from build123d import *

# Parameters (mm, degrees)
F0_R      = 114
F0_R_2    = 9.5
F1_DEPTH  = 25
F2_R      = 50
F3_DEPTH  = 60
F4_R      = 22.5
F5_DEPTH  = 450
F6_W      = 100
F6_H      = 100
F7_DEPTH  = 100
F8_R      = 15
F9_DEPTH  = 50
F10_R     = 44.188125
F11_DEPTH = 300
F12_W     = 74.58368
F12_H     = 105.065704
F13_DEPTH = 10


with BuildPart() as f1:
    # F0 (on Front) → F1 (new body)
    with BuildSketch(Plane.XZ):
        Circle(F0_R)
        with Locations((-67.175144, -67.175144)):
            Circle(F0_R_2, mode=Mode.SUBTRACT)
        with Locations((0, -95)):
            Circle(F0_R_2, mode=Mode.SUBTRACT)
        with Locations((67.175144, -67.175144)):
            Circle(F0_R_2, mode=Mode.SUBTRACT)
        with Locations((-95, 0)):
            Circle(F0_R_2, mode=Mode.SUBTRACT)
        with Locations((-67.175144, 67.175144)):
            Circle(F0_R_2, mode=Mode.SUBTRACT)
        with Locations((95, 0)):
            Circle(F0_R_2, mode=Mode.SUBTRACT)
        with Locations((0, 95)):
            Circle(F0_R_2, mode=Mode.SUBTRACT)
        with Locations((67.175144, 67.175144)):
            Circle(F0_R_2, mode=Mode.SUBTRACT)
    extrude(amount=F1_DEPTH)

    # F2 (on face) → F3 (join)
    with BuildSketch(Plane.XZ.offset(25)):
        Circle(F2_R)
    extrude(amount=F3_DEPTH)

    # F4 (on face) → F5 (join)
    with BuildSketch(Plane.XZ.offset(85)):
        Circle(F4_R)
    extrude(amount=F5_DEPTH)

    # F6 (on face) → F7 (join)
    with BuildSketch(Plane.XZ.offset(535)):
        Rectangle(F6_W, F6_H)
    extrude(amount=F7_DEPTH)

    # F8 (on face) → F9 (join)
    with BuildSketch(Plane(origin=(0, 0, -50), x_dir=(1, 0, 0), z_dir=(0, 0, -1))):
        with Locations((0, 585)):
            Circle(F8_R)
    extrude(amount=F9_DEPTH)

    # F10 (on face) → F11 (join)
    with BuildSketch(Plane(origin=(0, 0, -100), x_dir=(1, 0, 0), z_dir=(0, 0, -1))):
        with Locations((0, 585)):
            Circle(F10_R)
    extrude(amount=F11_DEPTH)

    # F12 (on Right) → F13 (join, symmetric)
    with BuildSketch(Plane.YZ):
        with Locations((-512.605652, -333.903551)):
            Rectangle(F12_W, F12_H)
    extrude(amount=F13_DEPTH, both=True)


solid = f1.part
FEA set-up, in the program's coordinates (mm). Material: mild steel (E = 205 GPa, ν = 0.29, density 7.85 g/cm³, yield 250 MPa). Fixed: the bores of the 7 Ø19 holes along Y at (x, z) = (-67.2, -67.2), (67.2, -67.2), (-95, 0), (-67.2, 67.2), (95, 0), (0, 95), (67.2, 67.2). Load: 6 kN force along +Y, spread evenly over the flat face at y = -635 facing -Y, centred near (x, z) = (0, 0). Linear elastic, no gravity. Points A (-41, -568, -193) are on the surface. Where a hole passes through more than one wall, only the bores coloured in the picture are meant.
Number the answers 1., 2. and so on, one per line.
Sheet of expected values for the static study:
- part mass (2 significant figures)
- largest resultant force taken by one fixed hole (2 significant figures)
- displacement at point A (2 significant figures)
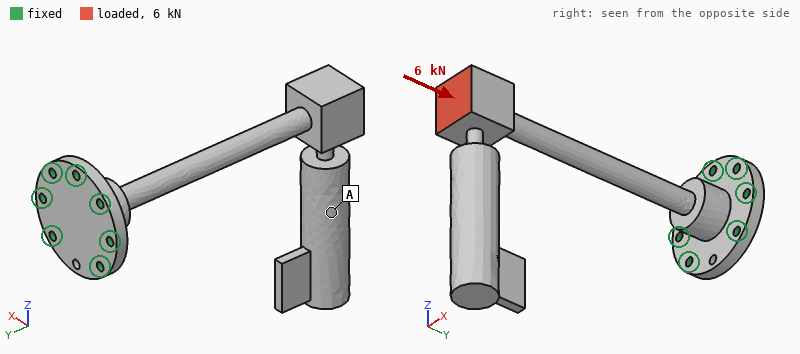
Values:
1. 41 kg
2. 1.2 kN
3. 11 µm
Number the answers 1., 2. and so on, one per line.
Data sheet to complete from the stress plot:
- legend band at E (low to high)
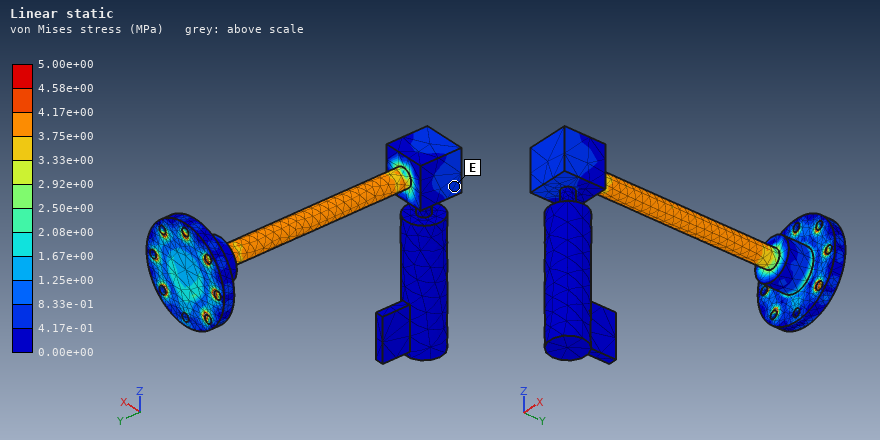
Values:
1. 4.17e-01 to 8.33e-01 MPa
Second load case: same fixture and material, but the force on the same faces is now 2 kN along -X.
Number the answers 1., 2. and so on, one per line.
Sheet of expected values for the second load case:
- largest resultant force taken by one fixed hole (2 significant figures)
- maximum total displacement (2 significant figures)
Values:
1. 4.2 kN
2. 2.9 mm
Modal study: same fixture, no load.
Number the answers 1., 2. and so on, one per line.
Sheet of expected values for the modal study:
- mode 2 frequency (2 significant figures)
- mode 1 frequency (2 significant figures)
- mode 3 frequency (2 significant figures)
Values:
1. 25 Hz
2. 25 Hz
3. 63 Hz
